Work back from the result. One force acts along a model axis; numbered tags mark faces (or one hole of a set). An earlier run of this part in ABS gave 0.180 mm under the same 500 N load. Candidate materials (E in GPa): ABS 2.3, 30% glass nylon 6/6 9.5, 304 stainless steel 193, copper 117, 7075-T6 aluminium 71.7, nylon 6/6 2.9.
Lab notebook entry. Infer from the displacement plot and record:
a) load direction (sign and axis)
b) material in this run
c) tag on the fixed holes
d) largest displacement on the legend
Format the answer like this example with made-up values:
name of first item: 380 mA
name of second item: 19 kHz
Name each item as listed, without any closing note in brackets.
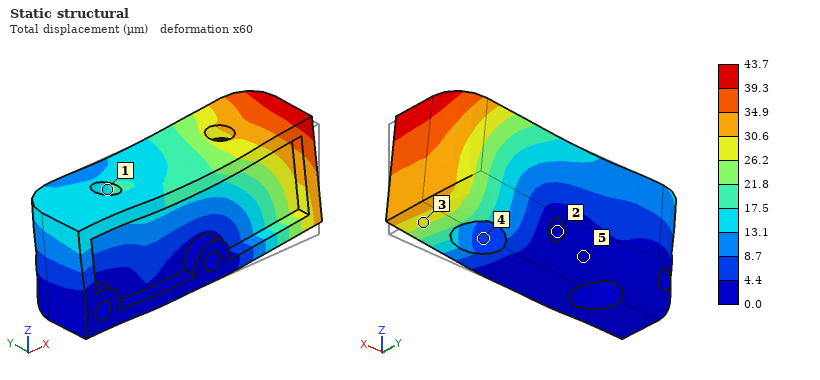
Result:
load direction: -X
material in this run: 30% glass nylon 6/6
tag on the fixed holes: 2
largest displacement on the legend: 43.7 µm
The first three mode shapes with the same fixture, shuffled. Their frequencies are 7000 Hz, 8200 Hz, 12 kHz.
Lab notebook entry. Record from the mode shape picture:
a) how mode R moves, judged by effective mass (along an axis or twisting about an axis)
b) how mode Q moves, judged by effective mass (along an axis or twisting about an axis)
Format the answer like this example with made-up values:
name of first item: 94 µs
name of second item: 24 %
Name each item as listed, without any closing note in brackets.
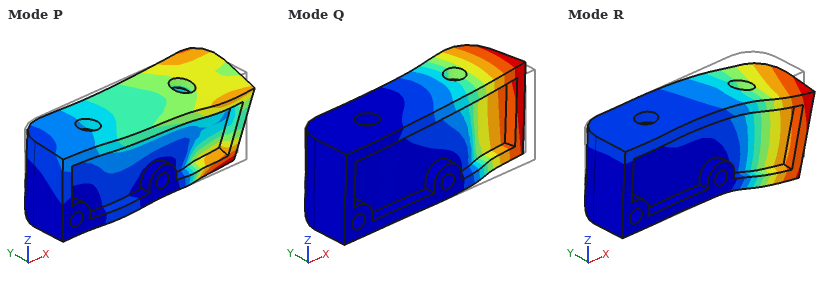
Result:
how mode R moves, judged by effective mass: along Z
how mode Q moves, judged by effective mass: along Y
